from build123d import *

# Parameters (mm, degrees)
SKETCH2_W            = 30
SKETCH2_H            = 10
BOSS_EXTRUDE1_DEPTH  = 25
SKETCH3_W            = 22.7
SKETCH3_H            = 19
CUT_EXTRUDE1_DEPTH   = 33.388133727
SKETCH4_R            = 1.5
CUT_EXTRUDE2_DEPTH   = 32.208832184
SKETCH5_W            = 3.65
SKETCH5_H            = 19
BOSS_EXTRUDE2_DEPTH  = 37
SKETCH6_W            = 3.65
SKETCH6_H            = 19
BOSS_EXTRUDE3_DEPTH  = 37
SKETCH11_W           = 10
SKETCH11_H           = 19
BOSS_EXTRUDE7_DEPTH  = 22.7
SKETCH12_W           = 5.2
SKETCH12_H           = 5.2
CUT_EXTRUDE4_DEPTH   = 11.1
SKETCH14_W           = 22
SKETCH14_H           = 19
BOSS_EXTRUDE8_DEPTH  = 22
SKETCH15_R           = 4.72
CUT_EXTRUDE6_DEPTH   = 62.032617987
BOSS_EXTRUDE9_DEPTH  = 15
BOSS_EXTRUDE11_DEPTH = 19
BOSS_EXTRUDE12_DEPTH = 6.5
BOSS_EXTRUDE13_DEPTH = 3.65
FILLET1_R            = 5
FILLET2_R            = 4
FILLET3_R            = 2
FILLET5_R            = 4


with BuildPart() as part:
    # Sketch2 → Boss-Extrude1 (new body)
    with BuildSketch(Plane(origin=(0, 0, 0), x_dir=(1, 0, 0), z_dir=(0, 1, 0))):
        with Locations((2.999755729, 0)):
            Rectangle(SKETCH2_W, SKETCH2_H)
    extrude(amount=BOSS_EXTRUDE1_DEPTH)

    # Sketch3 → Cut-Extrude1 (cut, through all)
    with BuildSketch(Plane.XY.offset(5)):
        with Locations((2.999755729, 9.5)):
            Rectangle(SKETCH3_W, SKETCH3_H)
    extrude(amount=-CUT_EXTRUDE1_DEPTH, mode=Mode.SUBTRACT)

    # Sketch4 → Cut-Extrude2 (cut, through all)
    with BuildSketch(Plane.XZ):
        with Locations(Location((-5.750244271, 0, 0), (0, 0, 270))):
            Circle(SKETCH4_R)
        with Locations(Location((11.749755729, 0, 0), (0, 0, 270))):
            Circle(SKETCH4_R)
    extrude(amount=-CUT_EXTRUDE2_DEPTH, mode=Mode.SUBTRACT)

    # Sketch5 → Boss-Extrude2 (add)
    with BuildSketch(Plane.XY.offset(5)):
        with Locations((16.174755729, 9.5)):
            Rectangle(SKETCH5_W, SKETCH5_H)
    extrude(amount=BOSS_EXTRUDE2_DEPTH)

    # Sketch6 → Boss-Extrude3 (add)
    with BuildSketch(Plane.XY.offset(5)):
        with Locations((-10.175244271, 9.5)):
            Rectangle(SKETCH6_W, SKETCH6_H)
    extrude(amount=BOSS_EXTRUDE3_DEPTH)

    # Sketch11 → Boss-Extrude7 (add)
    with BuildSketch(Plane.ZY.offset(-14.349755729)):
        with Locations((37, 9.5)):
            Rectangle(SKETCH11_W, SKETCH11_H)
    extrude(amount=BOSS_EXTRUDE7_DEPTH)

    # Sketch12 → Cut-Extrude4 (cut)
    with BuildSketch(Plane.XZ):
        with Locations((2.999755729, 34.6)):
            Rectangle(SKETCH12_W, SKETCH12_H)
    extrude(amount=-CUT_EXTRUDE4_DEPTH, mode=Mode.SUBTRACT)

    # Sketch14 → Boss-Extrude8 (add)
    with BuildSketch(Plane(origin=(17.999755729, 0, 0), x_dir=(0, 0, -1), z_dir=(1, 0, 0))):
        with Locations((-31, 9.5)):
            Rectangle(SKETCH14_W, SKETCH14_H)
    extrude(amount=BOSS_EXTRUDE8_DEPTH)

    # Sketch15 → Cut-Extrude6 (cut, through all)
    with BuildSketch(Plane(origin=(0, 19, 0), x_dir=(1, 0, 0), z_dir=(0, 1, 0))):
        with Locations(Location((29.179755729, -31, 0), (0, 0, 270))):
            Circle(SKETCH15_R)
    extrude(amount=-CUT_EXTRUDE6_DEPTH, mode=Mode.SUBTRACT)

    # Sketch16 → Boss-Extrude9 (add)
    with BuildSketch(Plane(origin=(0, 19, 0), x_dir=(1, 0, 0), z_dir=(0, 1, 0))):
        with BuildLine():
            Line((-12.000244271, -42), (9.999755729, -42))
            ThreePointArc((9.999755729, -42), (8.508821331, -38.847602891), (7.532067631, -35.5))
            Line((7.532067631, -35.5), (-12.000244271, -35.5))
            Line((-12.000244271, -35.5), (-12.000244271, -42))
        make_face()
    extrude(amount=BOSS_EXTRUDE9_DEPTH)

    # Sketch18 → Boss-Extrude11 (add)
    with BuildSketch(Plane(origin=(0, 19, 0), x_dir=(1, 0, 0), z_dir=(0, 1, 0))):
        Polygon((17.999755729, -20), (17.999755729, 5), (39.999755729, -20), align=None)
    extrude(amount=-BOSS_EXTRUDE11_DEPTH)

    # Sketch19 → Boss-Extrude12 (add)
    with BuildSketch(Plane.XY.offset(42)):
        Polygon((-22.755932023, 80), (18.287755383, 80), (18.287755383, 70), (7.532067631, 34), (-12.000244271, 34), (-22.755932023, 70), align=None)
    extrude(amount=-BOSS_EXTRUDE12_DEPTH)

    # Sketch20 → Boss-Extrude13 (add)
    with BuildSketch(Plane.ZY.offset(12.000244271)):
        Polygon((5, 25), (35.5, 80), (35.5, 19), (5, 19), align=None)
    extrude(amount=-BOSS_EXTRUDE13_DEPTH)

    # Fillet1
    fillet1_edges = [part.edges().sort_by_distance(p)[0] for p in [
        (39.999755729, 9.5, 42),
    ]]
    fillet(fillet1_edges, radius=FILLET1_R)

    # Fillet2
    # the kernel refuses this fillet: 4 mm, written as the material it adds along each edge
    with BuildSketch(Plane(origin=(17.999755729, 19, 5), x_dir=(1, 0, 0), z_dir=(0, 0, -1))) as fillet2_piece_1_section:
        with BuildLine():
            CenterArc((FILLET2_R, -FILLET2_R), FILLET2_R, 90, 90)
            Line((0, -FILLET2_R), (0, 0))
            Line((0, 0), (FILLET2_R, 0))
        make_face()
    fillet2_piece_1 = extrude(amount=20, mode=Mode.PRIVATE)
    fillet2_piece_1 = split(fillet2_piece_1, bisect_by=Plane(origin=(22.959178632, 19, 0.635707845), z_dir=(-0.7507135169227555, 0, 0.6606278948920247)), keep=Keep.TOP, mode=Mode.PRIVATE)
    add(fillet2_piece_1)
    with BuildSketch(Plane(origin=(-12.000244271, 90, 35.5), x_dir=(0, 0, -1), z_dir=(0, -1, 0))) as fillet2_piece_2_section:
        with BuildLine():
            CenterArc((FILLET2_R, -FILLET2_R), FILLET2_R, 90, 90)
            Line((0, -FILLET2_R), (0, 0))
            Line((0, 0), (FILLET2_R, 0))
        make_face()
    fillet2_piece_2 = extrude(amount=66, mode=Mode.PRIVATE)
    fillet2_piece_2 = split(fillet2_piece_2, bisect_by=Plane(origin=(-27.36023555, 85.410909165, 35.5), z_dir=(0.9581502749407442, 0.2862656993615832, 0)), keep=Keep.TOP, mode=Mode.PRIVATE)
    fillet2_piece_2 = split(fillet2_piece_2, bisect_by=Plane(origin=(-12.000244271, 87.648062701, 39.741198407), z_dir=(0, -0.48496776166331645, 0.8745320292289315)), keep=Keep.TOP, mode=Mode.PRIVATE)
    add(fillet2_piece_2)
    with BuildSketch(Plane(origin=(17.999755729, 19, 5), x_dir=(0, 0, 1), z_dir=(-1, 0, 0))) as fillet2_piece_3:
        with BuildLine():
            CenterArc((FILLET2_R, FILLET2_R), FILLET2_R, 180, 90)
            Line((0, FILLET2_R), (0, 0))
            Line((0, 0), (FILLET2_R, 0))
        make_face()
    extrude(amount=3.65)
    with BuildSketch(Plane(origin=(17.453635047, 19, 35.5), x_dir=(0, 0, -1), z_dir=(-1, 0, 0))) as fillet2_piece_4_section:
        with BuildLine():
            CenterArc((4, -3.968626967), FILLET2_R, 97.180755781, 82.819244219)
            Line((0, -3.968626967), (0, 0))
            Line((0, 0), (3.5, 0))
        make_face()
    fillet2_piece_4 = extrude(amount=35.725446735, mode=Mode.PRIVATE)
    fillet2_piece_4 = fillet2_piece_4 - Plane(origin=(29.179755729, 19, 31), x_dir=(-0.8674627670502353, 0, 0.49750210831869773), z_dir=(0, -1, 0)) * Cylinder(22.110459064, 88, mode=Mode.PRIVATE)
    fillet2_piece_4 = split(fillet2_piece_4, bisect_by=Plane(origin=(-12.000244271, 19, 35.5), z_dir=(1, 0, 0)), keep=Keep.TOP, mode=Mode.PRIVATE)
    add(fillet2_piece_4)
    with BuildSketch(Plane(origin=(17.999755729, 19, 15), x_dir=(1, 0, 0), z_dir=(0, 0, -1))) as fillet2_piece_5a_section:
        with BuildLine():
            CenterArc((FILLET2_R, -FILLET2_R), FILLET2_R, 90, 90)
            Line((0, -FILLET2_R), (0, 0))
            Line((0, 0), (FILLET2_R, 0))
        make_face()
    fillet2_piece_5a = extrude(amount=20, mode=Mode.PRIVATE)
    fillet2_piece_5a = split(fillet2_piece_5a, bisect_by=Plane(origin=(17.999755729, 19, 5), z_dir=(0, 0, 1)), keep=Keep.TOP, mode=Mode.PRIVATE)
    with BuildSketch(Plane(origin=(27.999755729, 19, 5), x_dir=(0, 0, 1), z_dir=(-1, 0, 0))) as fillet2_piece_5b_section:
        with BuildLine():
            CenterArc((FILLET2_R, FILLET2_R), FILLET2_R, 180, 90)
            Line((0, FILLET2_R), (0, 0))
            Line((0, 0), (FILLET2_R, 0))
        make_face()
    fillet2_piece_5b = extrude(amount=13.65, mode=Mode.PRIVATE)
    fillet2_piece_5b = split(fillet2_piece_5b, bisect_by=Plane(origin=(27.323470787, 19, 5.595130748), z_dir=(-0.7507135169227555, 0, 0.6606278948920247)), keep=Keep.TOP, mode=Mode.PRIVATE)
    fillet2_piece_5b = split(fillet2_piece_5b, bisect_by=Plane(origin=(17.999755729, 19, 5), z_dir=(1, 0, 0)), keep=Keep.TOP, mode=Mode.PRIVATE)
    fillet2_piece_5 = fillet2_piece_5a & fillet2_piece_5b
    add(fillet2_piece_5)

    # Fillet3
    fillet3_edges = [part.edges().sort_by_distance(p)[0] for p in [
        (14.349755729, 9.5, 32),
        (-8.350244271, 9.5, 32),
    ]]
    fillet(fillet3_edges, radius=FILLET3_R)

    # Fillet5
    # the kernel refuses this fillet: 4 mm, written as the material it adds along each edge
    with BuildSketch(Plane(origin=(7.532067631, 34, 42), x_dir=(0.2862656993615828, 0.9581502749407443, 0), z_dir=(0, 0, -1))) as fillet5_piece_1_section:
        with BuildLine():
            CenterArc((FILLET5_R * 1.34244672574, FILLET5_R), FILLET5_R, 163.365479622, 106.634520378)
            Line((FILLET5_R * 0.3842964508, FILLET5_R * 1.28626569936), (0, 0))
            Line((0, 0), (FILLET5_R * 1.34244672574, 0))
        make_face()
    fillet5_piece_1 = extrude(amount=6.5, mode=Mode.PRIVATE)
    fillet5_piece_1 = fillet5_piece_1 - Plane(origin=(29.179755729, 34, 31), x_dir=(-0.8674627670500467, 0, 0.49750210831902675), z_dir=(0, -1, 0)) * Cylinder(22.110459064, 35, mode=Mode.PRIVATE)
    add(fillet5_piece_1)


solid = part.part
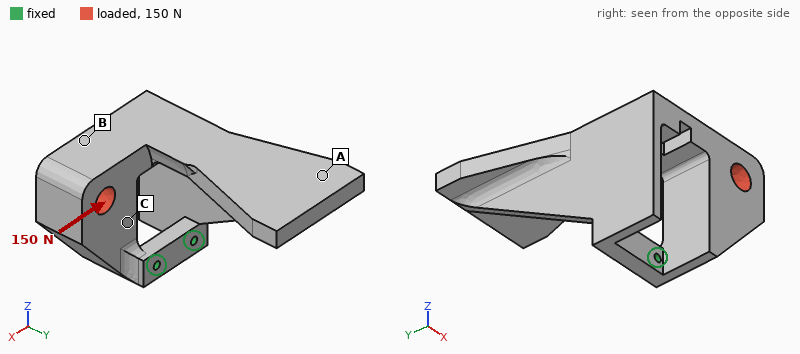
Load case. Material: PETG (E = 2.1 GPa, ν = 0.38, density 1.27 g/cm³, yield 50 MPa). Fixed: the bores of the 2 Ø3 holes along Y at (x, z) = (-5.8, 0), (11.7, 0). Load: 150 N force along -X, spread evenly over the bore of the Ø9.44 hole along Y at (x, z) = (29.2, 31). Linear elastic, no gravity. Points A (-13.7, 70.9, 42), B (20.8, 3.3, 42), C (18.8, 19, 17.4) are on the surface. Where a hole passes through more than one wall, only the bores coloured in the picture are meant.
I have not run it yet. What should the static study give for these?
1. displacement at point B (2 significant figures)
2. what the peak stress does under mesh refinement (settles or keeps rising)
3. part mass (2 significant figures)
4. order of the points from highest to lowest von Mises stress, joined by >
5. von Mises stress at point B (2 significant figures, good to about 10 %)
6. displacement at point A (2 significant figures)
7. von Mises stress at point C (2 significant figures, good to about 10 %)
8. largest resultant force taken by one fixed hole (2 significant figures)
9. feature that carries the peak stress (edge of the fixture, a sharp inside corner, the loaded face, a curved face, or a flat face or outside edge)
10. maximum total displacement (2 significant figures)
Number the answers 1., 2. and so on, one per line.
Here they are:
1. 0.86 mm
2. keeps rising
3. 52 g
4. B > C > A
5. 4.6 MPa
6. 0.24 mm
7. 2.4 MPa
8. 230 N
9. edge of the fixture
10. 0.99 mm
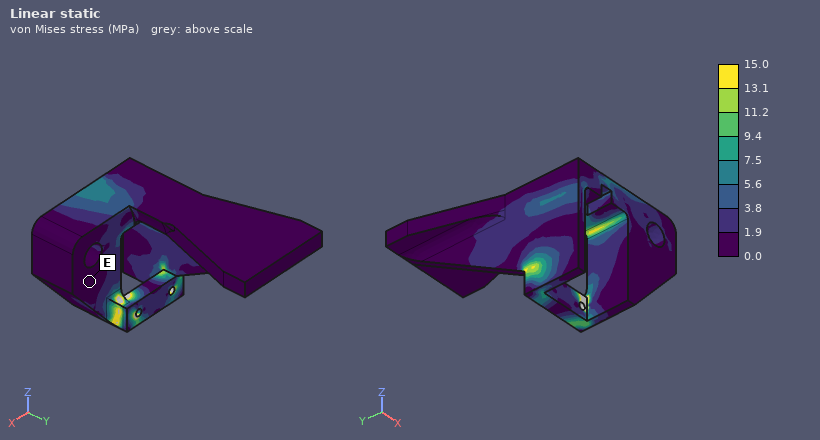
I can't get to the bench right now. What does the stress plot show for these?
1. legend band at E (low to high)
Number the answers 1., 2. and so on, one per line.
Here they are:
1. 0.0 to 1.9 MPa
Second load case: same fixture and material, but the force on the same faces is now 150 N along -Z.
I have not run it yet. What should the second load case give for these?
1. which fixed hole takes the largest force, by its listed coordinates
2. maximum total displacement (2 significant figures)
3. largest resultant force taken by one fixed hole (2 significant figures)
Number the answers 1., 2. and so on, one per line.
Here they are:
1. (11.7, 0)
2. 1.1 mm
3. 250 N
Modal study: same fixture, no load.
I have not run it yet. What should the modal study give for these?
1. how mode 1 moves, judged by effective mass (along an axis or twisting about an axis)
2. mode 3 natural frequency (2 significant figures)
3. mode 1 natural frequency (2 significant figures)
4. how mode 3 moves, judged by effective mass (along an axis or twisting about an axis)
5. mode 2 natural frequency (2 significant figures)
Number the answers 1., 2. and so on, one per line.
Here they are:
1. along Y
2. 420 Hz
3. 200 Hz
4. along X
5. 220 Hz
